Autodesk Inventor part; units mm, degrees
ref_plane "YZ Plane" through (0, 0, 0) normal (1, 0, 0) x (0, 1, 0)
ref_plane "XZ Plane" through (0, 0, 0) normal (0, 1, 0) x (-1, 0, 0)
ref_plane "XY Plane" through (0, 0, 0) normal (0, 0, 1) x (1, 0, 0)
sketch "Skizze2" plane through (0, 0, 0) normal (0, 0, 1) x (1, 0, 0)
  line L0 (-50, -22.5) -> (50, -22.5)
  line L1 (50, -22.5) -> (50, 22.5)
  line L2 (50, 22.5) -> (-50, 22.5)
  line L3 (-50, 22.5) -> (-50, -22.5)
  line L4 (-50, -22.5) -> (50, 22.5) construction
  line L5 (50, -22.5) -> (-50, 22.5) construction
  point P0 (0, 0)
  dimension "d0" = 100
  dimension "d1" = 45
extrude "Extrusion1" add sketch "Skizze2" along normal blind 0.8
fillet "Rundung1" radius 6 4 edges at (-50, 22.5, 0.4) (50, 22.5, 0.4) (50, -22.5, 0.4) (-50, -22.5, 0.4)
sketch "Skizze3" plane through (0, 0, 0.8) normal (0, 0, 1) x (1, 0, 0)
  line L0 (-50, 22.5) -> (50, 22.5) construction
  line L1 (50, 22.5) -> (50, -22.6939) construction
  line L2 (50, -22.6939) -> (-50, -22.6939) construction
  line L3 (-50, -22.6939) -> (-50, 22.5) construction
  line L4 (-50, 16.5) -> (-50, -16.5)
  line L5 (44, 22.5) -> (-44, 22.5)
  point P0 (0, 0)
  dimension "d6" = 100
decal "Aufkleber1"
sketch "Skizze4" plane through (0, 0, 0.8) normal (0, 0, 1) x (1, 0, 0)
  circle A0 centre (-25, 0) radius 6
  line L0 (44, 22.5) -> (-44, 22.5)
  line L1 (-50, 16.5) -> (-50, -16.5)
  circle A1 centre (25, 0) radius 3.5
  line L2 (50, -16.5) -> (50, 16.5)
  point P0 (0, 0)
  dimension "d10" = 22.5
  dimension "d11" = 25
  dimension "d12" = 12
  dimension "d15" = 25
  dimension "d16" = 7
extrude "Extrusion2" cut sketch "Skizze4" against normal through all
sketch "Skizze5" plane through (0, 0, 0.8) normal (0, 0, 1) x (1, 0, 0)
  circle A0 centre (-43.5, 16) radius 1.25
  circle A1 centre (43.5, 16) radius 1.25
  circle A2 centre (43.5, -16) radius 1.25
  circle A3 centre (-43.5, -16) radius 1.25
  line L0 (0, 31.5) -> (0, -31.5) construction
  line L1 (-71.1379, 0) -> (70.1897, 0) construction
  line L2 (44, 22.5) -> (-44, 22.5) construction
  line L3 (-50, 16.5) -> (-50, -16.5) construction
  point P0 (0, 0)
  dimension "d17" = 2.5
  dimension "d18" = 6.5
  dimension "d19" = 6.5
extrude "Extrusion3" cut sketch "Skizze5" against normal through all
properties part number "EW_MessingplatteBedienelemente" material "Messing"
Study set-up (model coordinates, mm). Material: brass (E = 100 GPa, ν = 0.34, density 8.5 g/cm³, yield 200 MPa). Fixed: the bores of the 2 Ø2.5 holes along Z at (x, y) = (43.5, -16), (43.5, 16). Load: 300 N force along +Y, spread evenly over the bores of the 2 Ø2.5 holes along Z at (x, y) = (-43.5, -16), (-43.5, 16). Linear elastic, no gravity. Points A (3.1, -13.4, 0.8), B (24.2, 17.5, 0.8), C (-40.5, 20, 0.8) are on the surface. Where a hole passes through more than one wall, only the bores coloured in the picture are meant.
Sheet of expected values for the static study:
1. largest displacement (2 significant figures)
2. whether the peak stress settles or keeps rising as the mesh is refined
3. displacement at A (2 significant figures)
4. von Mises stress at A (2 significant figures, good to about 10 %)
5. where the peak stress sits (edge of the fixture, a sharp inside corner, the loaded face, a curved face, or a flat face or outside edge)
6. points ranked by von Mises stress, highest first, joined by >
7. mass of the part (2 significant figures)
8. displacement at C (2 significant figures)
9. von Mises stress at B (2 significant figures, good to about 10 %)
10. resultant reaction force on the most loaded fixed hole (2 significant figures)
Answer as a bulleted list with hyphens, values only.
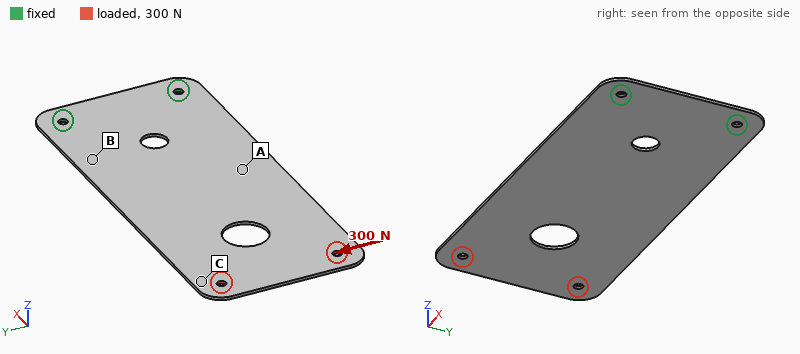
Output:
- 0.17 mm
- keeps rising
- 0.054 mm
- 33 MPa
- edge of the fixture
- B > A > C
- 29 g
- 0.15 mm
- 59 MPa
- 810 N
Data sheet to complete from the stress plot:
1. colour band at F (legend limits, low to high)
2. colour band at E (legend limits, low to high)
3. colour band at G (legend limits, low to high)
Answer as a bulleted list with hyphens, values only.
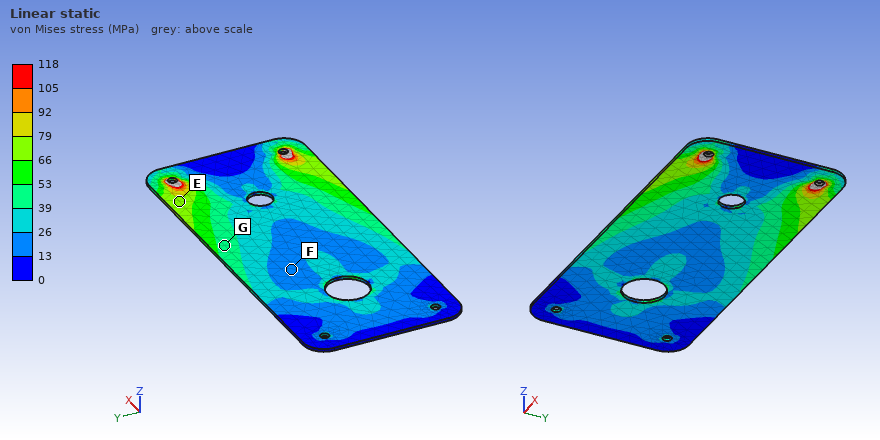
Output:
- 13 to 26 MPa
- 66 to 79 MPa
- 39 to 53 MPa
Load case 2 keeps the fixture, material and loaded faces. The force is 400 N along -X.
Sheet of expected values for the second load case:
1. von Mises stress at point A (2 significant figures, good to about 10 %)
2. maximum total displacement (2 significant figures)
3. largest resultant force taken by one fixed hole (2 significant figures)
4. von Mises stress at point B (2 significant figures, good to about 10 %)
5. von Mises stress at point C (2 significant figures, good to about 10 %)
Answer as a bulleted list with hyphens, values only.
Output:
- 11 MPa
- 14 µm
- 200 N
- 13 MPa
- 16 MPa
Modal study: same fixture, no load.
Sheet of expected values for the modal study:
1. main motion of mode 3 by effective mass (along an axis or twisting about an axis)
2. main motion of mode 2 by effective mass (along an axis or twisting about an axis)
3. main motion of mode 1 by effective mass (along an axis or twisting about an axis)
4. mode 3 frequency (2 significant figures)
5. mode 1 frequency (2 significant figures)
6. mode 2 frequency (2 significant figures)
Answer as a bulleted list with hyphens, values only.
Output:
- along Z
- twisting about X
- along Z
- 310 Hz
- 51 Hz
- 230 Hz
